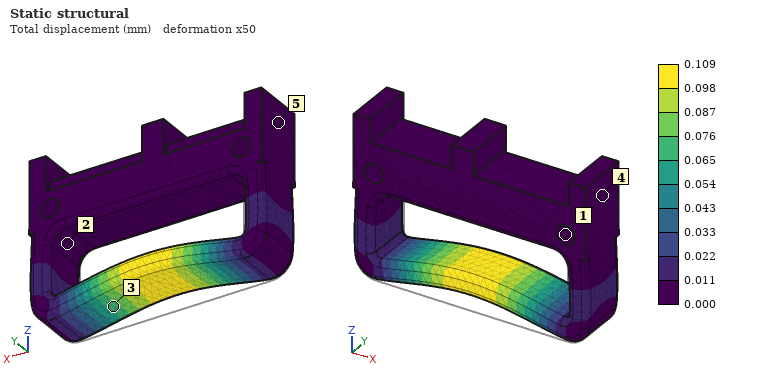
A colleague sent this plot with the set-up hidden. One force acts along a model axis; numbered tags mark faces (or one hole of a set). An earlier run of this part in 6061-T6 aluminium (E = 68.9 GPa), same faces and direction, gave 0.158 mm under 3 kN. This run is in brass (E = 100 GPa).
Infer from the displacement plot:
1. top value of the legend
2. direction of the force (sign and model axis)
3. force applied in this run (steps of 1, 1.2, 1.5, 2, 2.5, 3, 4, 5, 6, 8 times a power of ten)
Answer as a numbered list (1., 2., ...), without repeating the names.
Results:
1. 0.109 mm
2. +Z
3. 3 kN
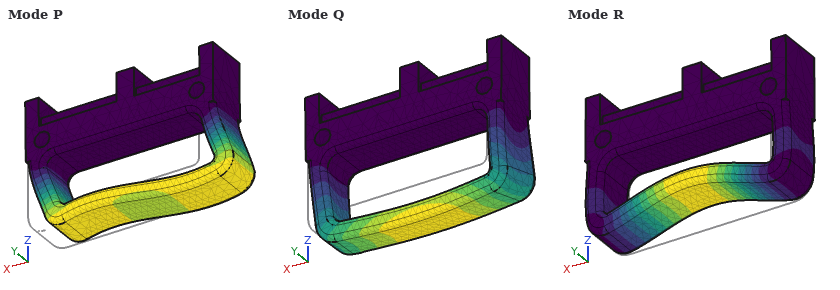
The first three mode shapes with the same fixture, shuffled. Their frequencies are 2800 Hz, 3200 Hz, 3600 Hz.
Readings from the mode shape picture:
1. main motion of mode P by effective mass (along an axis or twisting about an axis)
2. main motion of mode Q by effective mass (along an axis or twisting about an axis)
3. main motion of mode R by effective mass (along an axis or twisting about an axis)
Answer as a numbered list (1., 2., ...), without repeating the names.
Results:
1. along X
2. along Y
3. along Z
